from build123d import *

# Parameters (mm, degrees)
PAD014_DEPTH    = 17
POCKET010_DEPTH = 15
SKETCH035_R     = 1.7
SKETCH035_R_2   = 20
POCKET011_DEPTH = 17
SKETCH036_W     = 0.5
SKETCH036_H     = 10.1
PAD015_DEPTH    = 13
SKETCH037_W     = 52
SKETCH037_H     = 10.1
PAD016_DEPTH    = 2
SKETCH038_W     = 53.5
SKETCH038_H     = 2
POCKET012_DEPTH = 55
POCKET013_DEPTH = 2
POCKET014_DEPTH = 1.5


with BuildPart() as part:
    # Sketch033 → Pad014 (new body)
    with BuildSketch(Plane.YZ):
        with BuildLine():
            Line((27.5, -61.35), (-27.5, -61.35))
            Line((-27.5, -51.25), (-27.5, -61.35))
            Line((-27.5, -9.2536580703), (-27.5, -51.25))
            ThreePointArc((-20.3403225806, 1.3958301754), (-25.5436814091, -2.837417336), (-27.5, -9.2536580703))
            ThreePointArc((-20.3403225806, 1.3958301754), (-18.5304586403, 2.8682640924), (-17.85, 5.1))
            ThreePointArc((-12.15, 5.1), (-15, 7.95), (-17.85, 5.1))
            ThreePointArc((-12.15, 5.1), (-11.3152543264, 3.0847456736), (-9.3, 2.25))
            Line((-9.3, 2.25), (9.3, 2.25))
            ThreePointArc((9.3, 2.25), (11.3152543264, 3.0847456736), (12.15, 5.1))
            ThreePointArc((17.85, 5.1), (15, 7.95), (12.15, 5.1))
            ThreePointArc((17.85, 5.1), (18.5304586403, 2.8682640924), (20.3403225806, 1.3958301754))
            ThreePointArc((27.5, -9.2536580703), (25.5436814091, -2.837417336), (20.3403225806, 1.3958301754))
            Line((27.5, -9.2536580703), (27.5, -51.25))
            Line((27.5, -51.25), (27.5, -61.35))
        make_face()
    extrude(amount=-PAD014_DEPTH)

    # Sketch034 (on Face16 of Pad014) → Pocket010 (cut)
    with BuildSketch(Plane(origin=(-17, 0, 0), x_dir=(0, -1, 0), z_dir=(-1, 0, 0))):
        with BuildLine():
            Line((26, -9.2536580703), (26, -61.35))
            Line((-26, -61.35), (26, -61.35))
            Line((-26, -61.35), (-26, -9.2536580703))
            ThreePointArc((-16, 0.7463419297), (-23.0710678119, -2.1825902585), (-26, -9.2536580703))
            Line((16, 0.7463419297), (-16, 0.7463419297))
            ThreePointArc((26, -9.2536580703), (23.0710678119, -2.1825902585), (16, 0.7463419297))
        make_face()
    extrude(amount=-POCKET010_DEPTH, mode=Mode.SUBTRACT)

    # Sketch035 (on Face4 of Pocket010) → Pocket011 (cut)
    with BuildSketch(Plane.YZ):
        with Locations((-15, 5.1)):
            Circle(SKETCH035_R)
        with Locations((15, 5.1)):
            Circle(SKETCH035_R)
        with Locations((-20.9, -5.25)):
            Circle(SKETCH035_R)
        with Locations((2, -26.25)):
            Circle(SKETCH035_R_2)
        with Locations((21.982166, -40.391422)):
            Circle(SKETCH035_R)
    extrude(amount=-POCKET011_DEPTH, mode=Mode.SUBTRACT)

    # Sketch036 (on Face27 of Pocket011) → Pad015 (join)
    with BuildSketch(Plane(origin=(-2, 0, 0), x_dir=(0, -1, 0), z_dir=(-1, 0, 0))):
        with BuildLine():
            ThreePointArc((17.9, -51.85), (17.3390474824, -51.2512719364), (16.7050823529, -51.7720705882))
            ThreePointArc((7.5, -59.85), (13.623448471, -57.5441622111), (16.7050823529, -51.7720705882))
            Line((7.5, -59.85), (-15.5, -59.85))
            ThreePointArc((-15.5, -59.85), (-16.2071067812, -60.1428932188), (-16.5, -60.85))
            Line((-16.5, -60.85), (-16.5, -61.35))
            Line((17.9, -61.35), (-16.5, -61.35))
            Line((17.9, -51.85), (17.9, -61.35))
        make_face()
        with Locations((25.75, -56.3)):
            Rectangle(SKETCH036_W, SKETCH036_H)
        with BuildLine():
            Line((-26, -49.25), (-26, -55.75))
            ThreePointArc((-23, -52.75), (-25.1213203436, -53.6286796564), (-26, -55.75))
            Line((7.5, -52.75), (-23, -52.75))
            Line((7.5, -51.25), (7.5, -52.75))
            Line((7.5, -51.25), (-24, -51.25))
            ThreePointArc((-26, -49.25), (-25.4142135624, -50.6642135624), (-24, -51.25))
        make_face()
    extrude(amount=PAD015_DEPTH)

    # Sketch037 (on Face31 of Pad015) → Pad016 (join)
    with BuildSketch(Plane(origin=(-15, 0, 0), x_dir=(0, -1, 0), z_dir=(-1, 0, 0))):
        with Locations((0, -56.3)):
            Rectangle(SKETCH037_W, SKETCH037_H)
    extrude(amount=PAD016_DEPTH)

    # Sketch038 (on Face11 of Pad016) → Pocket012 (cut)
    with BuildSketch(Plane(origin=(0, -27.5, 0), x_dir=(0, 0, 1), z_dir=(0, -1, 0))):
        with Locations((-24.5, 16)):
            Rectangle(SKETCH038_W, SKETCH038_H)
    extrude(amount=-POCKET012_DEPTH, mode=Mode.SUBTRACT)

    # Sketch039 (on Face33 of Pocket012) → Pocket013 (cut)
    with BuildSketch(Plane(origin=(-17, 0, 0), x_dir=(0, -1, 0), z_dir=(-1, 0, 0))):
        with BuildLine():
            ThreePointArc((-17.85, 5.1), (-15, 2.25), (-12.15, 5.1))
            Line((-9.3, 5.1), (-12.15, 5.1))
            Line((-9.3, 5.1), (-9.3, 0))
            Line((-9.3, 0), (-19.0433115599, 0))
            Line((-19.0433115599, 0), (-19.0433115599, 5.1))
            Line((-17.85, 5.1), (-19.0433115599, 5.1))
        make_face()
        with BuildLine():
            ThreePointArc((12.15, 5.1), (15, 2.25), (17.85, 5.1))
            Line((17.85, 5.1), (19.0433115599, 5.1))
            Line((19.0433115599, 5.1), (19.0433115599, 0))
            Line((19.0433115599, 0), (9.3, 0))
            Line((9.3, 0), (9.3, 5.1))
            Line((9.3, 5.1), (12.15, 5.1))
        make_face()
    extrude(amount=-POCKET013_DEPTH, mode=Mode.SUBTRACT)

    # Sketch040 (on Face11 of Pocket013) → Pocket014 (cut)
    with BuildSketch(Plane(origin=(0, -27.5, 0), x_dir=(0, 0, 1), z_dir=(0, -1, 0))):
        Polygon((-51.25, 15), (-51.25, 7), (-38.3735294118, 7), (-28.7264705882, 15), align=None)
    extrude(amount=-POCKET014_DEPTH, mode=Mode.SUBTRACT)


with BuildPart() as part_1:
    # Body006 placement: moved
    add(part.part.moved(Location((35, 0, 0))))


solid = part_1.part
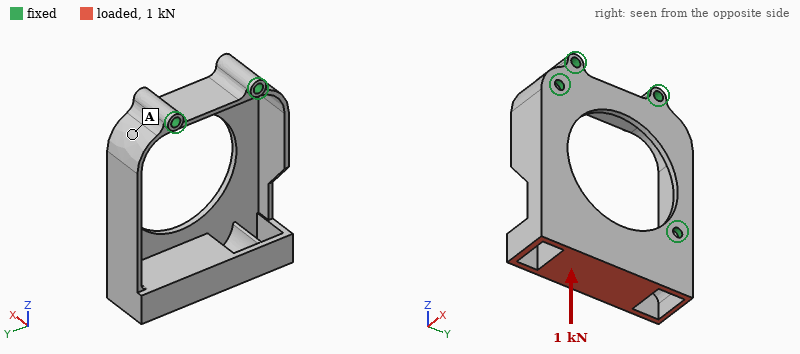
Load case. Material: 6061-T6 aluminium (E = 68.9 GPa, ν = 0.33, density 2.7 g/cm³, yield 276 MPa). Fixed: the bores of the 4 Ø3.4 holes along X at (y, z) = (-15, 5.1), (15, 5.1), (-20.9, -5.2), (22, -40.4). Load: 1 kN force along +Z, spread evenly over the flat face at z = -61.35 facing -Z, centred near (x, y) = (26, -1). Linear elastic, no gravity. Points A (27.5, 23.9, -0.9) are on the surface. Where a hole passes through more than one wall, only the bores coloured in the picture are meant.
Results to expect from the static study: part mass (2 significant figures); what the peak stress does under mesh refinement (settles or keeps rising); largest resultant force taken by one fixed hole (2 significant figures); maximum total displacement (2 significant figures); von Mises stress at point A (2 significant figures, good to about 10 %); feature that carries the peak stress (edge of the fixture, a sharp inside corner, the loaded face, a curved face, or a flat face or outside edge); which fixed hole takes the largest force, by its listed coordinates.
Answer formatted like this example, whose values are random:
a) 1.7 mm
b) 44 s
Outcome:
a) 30 g
b) keeps rising
c) 520 N
d) 0.23 mm
e) 18 MPa
f) a sharp inside corner
g) (-20.9, -5.2)
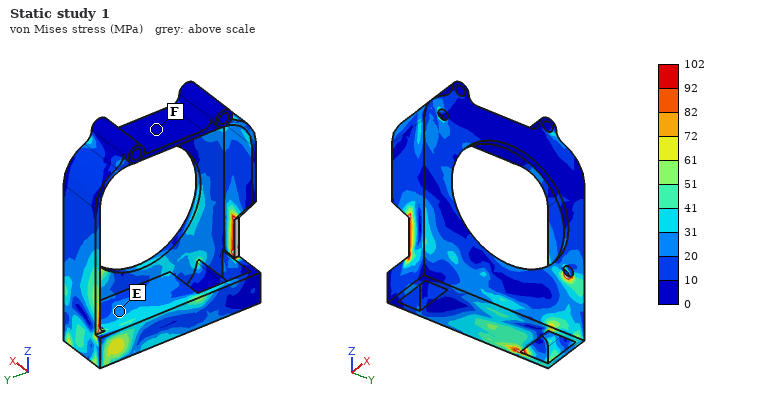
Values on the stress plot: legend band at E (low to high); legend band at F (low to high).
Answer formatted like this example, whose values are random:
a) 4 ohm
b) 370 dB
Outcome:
a) 20 to 31 MPa
b) 0 to 10 MPa
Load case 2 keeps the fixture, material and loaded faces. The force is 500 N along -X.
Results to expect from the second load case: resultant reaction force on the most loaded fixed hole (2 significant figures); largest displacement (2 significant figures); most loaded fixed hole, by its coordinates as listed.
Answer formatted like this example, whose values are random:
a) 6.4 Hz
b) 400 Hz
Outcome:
a) 680 N
b) 0.84 mm
c) (-20.9, -5.2)
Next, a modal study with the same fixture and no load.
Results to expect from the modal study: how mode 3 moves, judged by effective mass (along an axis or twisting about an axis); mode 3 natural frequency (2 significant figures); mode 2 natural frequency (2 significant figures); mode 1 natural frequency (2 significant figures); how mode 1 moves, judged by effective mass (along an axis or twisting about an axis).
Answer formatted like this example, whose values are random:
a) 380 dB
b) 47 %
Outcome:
a) along Y
b) 6100 Hz
c) 4200 Hz
d) 1300 Hz
e) along X
